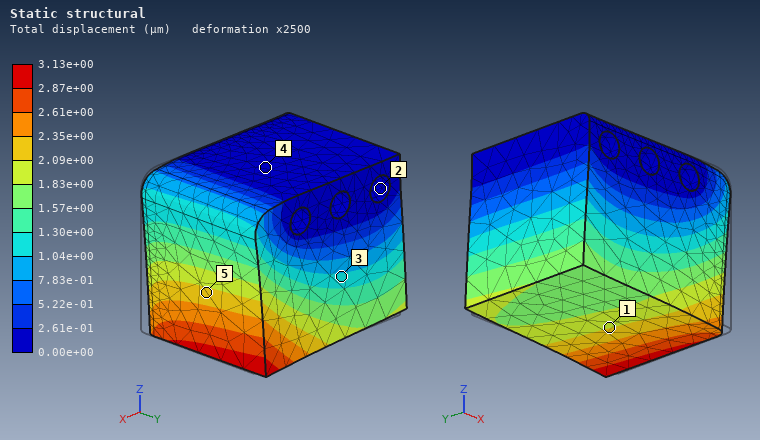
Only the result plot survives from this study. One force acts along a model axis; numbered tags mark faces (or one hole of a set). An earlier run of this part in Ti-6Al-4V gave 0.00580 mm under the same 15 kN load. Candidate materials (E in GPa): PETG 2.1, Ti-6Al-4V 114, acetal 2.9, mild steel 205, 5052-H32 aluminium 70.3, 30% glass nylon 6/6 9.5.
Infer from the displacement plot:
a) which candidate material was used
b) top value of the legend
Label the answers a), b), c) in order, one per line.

a) mild steel
b) 3.13e+00 µm
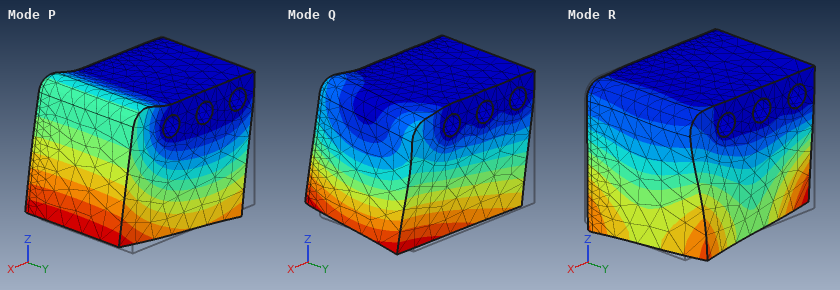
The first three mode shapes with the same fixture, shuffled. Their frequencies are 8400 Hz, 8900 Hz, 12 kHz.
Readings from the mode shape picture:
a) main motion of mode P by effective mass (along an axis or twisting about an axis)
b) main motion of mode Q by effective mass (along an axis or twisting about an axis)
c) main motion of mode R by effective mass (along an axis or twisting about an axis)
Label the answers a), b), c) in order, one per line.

a) along X
b) along Y
c) twisting about Z
